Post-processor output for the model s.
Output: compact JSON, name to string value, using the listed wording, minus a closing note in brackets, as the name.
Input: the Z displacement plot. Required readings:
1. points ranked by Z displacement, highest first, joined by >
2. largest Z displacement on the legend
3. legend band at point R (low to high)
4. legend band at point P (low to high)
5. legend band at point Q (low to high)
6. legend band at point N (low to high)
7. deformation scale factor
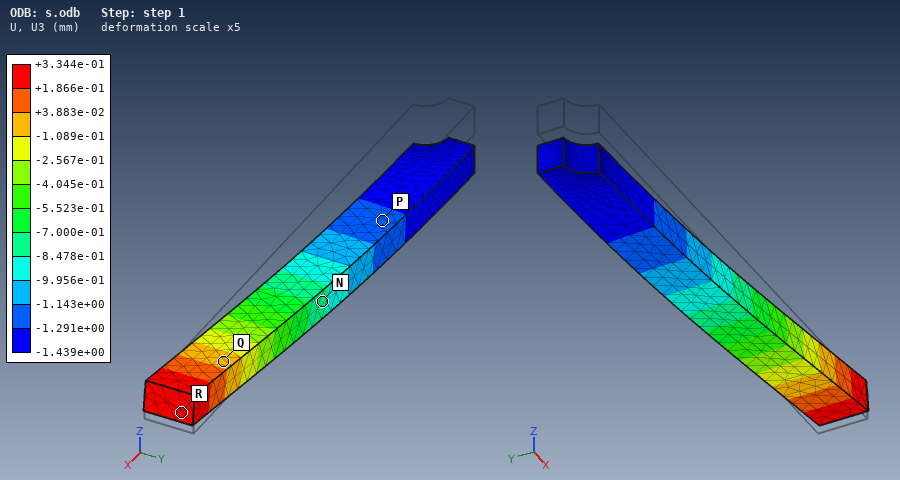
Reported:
{"points ranked by Z displacement, highest first, joined by >": "R > Q > N > P", "largest Z displacement on the legend": "+3.344e-01 mm", "legend band at point R": "+1.866e-01 to +3.344e-01 mm", "legend band at point P": "-1.291e+00 to -1.143e+00 mm", "legend band at point Q": "-1.089e-01 to +3.883e-02 mm", "legend band at point N": "-8.478e-01 to -7.000e-01 mm", "deformation scale factor": "5"}
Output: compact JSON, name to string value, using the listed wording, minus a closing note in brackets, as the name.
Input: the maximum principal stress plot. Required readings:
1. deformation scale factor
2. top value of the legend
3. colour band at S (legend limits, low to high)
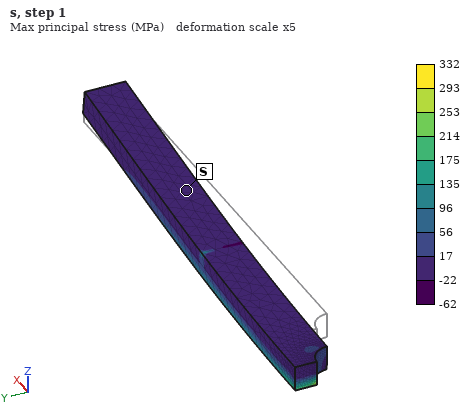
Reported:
{"deformation scale factor": "5", "top value of the legend": "332 MPa", "colour band at S": "-22 to 17 MPa"}
